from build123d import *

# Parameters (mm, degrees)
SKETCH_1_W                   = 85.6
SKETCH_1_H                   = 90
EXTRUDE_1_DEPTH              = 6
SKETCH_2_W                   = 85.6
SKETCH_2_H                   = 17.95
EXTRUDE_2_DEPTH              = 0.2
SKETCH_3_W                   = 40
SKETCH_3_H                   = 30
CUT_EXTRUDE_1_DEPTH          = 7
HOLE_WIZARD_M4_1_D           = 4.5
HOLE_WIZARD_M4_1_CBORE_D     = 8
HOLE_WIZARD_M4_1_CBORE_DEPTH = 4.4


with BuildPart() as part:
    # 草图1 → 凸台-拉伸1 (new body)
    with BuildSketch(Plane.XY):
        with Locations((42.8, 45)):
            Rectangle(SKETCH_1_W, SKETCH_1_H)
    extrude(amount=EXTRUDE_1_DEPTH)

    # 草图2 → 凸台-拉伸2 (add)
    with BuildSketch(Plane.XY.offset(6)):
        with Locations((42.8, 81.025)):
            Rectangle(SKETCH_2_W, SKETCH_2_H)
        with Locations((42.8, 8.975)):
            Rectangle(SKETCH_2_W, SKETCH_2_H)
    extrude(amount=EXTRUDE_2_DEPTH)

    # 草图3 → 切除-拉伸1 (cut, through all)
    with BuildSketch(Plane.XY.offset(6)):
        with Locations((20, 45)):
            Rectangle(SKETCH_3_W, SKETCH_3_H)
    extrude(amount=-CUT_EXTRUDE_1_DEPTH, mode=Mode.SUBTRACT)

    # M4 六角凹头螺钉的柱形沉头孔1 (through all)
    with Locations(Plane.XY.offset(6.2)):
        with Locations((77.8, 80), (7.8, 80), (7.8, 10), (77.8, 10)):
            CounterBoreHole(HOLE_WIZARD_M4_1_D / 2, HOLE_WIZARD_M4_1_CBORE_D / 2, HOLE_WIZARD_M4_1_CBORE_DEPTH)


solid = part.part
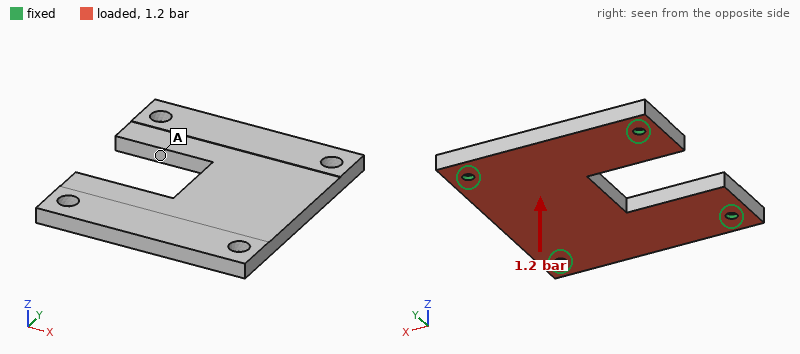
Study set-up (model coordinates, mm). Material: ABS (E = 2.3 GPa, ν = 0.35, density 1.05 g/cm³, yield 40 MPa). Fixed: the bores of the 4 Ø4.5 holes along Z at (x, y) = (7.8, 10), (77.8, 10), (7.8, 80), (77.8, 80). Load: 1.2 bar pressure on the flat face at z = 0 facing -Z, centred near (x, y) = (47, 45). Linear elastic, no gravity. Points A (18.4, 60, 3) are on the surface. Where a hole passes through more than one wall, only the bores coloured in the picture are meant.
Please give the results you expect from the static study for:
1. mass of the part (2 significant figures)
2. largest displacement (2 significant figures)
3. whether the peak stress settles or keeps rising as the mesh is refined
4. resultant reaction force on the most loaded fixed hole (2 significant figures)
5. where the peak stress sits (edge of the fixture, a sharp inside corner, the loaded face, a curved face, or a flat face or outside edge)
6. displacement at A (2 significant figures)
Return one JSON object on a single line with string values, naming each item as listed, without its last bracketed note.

{"mass of the part": "41 g", "largest displacement": "0.93 mm", "whether the peak stress settles or keeps rising as the mesh is refined": "keeps rising", "resultant reaction force on the most loaded fixed hole": "390 N", "where the peak stress sits": "edge of the fixture", "displacement at A": "0.57 mm"}
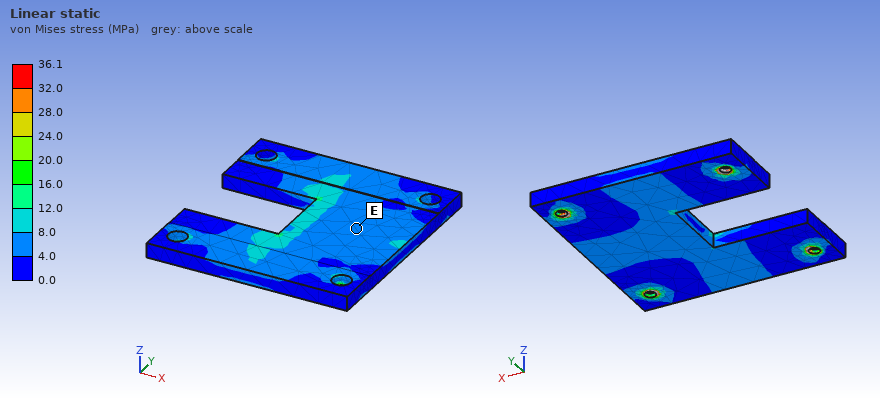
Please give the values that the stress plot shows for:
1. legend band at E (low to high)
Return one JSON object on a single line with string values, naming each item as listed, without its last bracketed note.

{"legend band at E": "4.0 to 8.0 MPa"}
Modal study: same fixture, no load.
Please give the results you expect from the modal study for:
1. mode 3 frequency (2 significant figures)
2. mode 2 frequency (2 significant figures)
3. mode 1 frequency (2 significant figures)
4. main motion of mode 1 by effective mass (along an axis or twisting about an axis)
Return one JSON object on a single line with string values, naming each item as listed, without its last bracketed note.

{"mode 3 frequency": "1500 Hz", "mode 2 frequency": "1400 Hz", "mode 1 frequency": "940 Hz", "main motion of mode 1 by effective mass": "along Z"}
